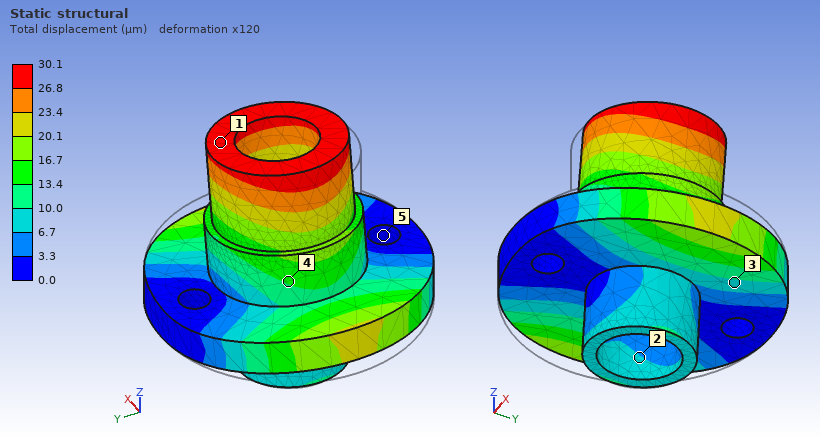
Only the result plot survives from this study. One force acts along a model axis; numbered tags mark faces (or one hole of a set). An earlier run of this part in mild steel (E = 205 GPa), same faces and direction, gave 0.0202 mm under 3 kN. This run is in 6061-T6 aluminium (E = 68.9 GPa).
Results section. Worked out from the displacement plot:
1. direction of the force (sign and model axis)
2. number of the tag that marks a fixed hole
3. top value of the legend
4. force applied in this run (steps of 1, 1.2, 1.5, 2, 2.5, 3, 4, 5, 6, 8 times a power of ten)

+X
5
30.1 µm
1.5 kN
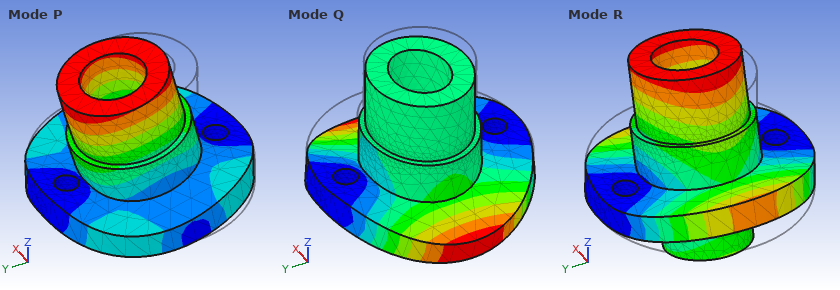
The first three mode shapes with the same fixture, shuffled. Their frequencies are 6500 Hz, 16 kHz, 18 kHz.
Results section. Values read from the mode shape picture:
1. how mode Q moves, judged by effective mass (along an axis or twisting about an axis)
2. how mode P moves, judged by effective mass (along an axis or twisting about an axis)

along Z
along Y
